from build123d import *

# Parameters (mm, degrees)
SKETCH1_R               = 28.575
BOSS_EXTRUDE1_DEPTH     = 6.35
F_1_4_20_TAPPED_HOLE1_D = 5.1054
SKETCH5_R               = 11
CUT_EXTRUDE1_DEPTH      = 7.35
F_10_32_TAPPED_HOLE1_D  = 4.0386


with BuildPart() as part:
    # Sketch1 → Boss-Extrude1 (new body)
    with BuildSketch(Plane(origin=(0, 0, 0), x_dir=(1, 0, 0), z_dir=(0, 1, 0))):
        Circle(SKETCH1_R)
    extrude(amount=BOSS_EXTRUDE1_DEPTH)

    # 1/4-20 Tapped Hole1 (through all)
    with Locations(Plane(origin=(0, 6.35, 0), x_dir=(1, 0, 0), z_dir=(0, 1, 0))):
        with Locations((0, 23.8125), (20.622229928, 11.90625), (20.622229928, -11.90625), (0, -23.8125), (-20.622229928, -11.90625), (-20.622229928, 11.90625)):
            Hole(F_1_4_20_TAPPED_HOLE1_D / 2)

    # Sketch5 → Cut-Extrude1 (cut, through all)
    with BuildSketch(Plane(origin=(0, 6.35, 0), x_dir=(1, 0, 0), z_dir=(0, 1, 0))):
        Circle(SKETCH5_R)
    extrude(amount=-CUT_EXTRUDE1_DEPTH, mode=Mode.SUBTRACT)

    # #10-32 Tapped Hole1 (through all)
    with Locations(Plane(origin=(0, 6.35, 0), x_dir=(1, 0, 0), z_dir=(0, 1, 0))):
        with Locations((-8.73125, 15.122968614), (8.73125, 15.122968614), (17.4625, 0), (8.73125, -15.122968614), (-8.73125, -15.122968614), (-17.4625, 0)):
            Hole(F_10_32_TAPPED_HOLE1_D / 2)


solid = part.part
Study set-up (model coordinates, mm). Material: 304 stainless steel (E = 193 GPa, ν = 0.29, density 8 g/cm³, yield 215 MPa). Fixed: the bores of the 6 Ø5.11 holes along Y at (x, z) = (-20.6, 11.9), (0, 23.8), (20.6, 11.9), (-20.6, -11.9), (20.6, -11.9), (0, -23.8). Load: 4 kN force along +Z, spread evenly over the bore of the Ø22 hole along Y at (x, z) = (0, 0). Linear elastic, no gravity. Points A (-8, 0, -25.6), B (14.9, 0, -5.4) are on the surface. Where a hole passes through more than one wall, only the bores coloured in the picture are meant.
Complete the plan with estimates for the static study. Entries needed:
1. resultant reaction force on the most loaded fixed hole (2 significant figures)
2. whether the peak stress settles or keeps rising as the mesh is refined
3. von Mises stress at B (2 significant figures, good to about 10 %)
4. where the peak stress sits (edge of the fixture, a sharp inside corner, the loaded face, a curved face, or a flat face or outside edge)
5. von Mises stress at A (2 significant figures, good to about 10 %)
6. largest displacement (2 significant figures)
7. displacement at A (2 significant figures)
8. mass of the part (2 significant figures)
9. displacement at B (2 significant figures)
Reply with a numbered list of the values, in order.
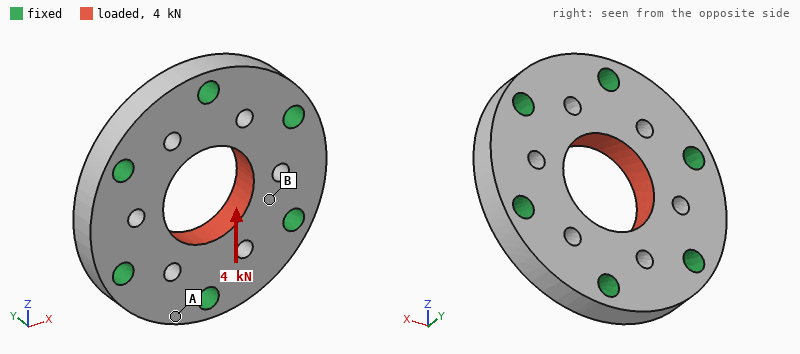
1. 960 N
2. keeps rising
3. 9.3 MPa
4. edge of the fixture
5. 2.8 MPa
6. 0.91 µm
7. 0.28 µm
8. 100 g
9. 0.40 µm
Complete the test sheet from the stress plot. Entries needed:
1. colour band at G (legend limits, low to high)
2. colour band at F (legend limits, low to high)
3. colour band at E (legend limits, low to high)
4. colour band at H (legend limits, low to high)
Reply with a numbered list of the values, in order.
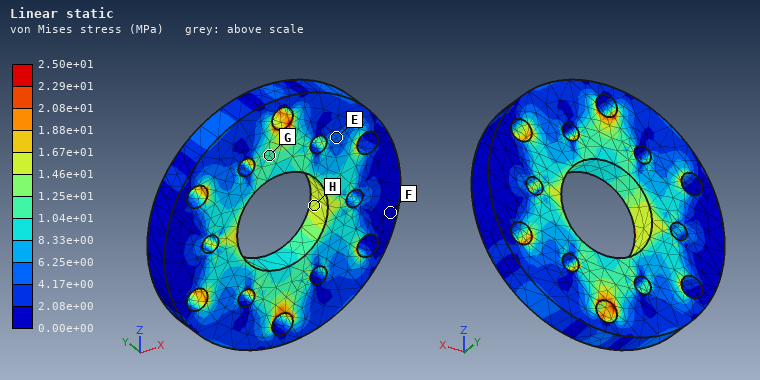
1. 1.04e+01 to 1.25e+01 MPa
2. 0.00e+00 to 2.08e+00 MPa
3. 4.17e+00 to 6.25e+00 MPa
4. 1.46e+01 to 1.67e+01 MPa
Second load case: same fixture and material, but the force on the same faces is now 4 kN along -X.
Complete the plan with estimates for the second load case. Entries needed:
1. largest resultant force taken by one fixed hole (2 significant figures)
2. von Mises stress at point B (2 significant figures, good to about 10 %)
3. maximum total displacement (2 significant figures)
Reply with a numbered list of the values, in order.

1. 850 N
2. 9.4 MPa
3. 0.92 µm
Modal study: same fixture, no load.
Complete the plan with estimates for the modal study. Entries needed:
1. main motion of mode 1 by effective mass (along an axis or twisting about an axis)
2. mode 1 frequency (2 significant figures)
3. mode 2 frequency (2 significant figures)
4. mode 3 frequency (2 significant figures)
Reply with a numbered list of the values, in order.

1. along Y
2. 31 kHz
3. 38 kHz
4. 38 kHz
